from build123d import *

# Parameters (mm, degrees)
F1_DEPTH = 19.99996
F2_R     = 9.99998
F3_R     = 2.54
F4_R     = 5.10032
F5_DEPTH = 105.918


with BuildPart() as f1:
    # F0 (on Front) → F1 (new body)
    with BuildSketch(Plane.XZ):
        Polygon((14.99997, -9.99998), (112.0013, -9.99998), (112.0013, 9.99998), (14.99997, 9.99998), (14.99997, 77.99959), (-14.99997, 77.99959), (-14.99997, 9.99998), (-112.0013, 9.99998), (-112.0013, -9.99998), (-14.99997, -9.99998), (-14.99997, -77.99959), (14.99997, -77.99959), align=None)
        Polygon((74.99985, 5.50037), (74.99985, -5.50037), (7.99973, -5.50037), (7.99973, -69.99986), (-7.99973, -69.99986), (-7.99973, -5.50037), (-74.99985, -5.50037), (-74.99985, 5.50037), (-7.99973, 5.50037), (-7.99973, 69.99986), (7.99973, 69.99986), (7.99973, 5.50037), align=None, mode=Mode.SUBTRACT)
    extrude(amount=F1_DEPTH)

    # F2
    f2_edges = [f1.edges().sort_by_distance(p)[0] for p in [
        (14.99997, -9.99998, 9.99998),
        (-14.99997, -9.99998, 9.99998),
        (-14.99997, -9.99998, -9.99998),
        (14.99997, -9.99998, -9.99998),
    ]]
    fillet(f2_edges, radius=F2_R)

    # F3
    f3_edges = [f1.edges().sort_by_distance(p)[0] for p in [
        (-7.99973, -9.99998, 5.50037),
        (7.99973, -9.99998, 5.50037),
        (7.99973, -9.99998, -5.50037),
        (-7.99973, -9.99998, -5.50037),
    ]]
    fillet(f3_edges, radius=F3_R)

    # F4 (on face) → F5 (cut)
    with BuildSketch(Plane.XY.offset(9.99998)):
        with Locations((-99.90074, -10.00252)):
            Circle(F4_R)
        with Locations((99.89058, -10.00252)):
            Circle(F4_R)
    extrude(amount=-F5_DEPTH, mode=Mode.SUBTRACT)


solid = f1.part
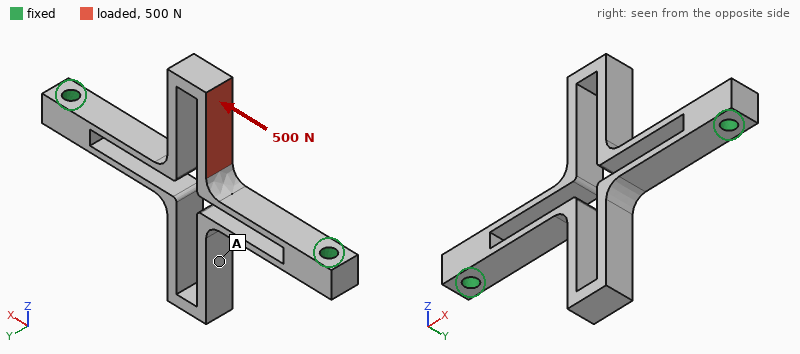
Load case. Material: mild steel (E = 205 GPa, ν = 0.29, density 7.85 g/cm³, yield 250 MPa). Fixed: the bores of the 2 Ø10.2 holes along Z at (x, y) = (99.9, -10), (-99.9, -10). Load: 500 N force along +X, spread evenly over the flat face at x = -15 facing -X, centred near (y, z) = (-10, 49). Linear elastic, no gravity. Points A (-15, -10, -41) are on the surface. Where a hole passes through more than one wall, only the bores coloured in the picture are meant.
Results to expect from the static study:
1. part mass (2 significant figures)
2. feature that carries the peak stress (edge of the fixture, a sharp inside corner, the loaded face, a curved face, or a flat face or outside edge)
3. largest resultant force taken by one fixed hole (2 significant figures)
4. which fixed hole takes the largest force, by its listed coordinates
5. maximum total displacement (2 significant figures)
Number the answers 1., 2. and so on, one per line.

1. 750 g
2. a curved face
3. 370 N
4. (-99.9, -10)
5. 0.19 mm
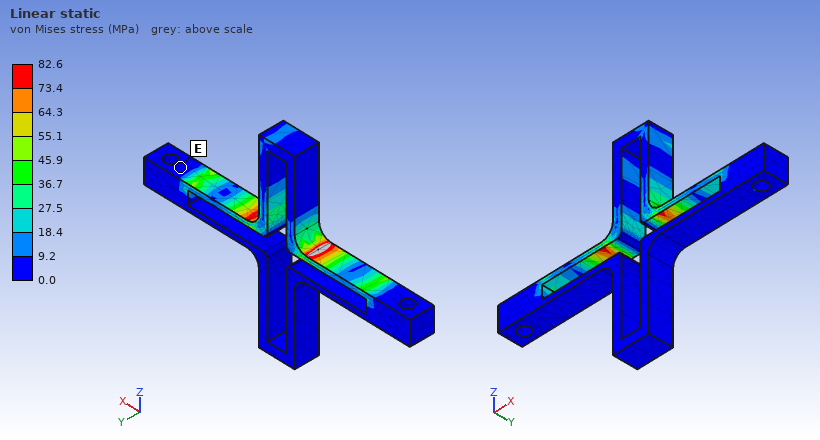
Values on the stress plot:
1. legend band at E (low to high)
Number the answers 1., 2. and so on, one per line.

1. 0.0 to 9.2 MPa
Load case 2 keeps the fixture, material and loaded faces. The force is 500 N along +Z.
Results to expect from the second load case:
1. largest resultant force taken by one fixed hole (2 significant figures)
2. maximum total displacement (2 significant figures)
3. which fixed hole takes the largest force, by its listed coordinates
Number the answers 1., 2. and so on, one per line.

1. 370 N
2. 0.21 mm
3. (-99.9, -10)
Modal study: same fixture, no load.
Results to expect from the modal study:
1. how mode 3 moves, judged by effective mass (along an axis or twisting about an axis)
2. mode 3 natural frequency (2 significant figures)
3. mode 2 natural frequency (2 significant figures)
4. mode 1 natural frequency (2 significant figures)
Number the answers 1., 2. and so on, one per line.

1. along Z
2. 590 Hz
3. 340 Hz
4. 340 Hz
